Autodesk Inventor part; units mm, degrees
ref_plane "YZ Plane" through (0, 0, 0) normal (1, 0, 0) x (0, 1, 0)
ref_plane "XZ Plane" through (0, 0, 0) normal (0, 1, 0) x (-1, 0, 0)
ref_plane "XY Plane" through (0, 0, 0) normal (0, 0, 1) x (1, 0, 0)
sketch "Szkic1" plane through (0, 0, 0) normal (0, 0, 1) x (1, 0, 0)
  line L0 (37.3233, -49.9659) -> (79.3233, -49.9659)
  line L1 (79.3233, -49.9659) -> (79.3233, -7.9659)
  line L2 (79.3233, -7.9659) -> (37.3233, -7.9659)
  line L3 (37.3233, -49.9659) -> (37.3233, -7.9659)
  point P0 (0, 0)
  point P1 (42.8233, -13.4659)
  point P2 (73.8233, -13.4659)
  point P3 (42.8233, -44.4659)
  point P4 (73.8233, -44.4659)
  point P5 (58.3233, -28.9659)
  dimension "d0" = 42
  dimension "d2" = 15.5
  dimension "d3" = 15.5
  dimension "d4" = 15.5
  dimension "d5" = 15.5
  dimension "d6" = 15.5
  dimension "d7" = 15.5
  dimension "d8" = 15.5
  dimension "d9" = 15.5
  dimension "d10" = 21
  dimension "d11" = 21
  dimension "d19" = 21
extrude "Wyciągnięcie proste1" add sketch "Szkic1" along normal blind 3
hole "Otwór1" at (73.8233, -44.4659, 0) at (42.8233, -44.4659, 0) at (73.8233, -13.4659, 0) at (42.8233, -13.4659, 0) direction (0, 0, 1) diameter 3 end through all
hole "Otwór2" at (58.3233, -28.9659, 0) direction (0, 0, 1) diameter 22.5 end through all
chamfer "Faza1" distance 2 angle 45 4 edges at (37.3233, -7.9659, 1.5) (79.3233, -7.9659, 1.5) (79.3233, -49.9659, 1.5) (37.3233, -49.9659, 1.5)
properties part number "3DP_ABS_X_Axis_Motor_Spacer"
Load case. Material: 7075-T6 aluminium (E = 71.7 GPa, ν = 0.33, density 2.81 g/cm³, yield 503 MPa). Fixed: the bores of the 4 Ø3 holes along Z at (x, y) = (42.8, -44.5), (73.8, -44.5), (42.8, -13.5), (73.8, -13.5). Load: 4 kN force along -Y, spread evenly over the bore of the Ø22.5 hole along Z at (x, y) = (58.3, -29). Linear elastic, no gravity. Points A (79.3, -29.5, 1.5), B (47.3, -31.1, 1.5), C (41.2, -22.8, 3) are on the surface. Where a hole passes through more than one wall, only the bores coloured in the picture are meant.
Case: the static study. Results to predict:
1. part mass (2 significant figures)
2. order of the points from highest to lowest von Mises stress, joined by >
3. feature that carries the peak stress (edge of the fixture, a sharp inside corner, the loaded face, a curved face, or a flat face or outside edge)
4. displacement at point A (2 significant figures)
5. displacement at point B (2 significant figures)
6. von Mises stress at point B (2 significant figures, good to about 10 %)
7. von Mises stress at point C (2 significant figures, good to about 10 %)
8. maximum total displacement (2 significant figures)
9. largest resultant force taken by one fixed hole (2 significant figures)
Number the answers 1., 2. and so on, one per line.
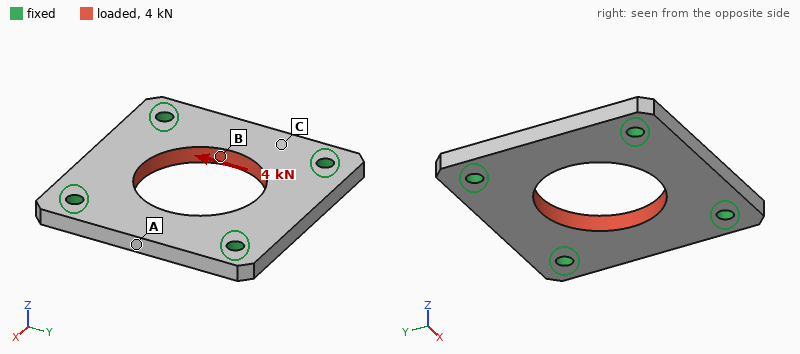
1. 11 g
2. B > C > A
3. edge of the fixture
4. 3.1 µm
5. 5.3 µm
6. 34 MPa
7. 19 MPa
8. 12 µm
9. 1.0 kN
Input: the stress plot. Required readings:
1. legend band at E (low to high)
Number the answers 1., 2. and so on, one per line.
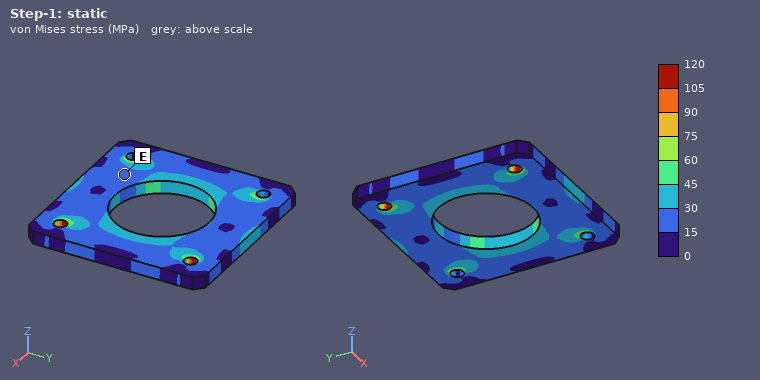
1. 15 to 30 MPa
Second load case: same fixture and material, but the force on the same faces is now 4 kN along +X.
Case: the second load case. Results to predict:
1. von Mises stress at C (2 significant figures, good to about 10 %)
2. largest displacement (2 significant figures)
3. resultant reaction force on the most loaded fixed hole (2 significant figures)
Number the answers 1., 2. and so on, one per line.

1. 21 MPa
2. 12 µm
3. 1.0 kN
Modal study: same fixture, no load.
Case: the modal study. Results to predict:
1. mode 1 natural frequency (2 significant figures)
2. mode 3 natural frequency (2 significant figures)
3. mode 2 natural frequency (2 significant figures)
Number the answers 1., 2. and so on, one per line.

1. 16 kHz
2. 17 kHz
3. 16 kHz
